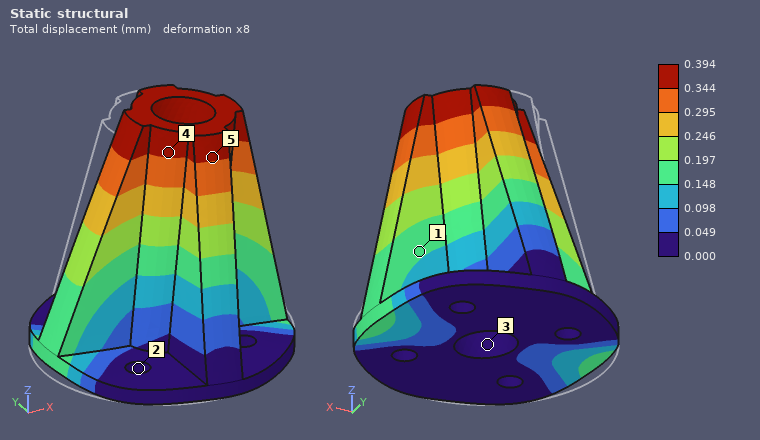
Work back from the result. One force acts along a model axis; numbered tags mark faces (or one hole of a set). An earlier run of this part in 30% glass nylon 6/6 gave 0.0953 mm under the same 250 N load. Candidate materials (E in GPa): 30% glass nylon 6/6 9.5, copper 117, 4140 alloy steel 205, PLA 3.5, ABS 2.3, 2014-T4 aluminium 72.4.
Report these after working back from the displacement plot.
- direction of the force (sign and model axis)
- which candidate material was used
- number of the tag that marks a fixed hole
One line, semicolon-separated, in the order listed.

+X; ABS; 2
